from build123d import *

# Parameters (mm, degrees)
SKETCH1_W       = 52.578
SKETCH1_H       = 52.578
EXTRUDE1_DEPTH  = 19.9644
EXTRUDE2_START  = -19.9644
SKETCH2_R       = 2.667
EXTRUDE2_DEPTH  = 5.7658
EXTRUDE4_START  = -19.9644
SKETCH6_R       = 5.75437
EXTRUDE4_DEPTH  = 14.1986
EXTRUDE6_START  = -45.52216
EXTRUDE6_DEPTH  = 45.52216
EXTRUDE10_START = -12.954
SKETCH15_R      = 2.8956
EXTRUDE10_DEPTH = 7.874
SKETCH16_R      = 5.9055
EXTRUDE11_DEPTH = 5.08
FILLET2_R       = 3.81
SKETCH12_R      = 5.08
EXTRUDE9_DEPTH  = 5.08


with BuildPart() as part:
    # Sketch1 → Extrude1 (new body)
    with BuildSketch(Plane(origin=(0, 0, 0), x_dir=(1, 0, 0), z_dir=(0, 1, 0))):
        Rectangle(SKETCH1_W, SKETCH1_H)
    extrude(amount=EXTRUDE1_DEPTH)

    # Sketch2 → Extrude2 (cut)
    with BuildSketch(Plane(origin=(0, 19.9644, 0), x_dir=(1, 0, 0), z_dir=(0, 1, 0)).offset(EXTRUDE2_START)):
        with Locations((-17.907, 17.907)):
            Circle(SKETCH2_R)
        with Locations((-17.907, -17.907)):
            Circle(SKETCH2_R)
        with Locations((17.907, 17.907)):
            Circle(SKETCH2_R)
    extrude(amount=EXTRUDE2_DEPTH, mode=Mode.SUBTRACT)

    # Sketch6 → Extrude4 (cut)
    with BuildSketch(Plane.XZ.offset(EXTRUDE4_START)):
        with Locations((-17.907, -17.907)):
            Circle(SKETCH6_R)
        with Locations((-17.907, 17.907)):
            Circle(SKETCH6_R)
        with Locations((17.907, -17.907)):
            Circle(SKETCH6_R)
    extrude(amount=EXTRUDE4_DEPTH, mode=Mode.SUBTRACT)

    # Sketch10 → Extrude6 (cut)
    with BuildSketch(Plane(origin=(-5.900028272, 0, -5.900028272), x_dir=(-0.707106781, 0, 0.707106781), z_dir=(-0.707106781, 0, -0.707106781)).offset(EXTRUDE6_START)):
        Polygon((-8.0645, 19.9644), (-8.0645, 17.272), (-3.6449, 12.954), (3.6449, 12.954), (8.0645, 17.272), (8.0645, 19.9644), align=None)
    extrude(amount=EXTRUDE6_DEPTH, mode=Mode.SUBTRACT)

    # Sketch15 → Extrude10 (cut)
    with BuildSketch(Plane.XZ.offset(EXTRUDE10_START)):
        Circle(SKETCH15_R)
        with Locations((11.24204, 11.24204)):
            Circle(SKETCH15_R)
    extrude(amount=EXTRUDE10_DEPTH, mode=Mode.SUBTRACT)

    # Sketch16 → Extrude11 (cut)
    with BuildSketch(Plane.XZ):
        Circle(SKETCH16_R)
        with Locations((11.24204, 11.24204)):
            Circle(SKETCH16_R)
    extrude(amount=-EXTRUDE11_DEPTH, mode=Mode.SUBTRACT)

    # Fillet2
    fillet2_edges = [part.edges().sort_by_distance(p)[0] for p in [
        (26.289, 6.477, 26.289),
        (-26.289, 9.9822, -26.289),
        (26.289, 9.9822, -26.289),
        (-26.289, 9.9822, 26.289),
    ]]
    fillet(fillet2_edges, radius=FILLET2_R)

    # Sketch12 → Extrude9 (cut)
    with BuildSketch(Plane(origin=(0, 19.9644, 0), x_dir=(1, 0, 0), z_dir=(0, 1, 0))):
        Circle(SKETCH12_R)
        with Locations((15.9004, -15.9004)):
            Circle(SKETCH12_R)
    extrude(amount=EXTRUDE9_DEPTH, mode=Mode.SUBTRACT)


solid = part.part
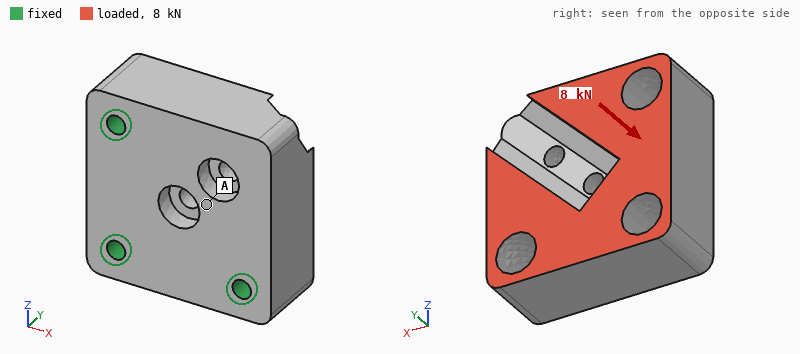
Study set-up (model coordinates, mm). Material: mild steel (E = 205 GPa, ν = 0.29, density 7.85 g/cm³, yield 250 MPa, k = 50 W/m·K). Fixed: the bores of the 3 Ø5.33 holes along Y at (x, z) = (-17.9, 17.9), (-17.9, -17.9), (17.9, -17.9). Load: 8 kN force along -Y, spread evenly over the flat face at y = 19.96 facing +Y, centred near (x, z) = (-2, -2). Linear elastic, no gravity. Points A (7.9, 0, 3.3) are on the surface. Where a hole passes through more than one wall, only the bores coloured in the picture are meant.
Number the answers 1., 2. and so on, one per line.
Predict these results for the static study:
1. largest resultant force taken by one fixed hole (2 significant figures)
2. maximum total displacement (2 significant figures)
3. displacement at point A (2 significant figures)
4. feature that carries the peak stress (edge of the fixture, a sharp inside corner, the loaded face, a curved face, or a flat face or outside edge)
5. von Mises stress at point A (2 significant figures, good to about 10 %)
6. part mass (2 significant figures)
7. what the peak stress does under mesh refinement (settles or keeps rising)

1. 3.5 kN
2. 12 µm
3. 5.7 µm
4. edge of the fixture
5. 13 MPa
6. 350 g
7. keeps rising
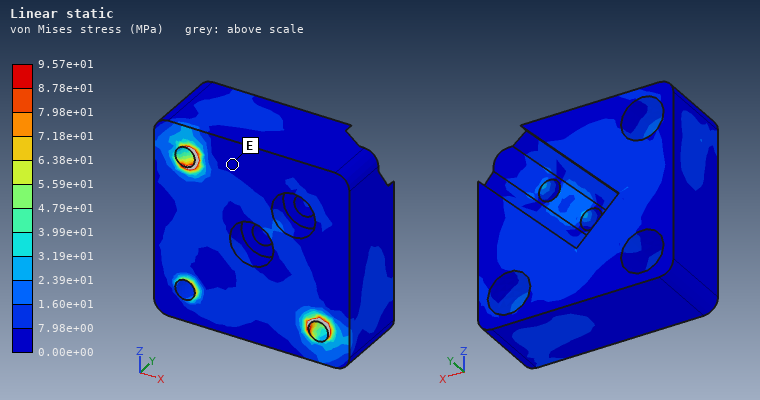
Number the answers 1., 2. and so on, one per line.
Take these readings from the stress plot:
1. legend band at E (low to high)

1. 0.00e+00 to 7.98e+00 MPa
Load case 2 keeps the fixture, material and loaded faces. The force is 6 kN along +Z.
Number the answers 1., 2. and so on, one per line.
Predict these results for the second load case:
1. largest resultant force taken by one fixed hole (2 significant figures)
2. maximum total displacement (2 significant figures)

1. 3.5 kN
2. 11 µm
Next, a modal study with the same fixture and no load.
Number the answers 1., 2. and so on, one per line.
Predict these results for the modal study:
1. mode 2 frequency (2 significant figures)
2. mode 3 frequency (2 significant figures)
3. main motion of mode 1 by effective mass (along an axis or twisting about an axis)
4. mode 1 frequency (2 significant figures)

1. 16 kHz
2. 18 kHz
3. along Y
4. 7300 Hz
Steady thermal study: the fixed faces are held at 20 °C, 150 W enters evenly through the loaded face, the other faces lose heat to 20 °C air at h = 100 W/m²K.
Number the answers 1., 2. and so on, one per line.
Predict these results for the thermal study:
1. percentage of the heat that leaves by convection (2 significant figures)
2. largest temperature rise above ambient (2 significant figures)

1. 24 %
2. 57 K
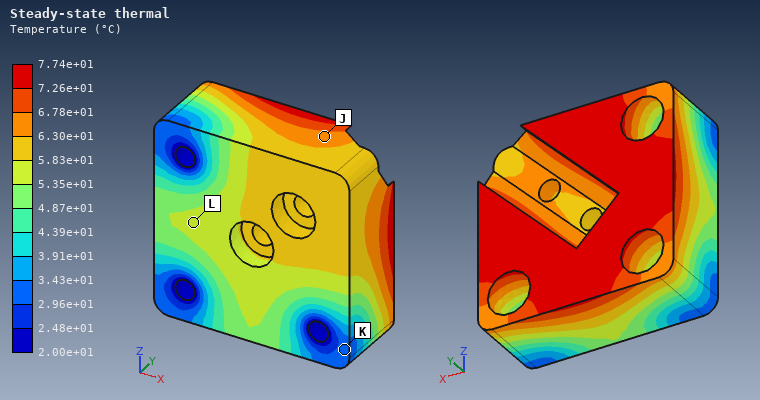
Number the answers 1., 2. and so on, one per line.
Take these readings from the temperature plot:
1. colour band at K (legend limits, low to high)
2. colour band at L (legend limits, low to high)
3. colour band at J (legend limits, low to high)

1. 2.96e+01 to 3.43e+01 °C
2. 5.35e+01 to 5.83e+01 °C
3. 6.30e+01 to 6.78e+01 °C
